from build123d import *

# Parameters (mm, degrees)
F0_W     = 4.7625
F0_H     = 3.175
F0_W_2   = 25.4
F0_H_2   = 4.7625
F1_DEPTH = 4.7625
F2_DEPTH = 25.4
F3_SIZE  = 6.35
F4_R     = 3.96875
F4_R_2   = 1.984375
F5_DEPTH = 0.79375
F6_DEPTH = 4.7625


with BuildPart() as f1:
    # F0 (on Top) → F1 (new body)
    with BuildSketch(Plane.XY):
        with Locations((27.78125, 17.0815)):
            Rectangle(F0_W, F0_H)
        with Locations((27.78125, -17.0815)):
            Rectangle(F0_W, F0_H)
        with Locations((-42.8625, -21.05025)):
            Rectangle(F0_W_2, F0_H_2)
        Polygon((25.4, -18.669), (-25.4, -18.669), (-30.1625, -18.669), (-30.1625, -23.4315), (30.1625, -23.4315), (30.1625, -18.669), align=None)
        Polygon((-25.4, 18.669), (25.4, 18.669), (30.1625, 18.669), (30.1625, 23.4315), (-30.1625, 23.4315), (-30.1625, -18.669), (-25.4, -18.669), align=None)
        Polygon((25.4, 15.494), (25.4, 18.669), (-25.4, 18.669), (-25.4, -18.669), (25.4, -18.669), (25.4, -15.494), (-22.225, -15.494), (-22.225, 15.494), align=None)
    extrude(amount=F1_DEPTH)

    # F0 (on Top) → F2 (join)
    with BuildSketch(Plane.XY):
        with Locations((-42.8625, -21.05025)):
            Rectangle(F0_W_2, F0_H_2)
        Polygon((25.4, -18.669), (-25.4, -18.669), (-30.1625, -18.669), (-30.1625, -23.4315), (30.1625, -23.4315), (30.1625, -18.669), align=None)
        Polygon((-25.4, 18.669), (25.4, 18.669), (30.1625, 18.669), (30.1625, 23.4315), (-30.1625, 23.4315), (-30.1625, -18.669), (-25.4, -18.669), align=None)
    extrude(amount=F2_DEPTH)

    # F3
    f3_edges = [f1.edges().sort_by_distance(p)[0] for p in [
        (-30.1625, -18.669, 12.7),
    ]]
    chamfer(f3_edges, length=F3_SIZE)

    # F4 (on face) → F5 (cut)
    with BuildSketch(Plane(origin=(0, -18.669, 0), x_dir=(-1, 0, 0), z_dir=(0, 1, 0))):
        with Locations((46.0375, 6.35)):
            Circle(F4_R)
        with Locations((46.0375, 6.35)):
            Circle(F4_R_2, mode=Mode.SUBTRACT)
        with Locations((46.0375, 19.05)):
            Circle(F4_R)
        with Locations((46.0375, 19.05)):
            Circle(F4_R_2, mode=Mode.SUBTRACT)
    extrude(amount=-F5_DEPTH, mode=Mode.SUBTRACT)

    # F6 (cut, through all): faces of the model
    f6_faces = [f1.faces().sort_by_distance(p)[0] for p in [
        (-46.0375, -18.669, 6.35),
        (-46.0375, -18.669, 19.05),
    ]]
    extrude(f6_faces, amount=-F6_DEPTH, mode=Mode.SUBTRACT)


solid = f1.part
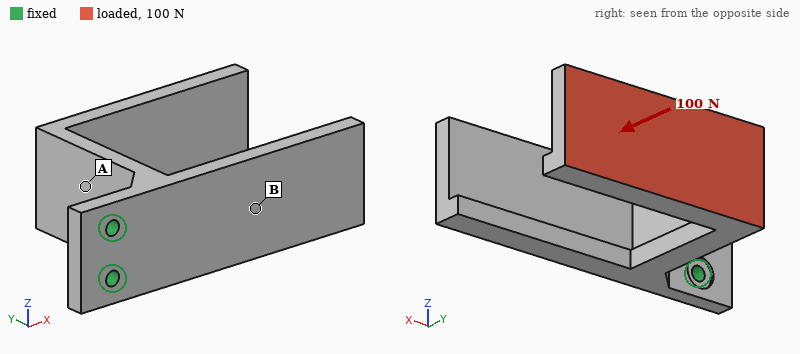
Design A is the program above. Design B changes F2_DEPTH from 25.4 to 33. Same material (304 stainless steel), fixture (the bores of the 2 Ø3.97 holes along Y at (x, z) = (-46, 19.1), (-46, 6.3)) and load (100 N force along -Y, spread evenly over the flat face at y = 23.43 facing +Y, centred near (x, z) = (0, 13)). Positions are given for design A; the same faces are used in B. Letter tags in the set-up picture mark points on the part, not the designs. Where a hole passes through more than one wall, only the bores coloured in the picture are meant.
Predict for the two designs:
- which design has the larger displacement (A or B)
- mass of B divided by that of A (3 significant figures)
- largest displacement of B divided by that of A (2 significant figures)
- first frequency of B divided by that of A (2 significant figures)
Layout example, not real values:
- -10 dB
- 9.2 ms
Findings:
- A
- 1.28
- 0.85
- 0.97
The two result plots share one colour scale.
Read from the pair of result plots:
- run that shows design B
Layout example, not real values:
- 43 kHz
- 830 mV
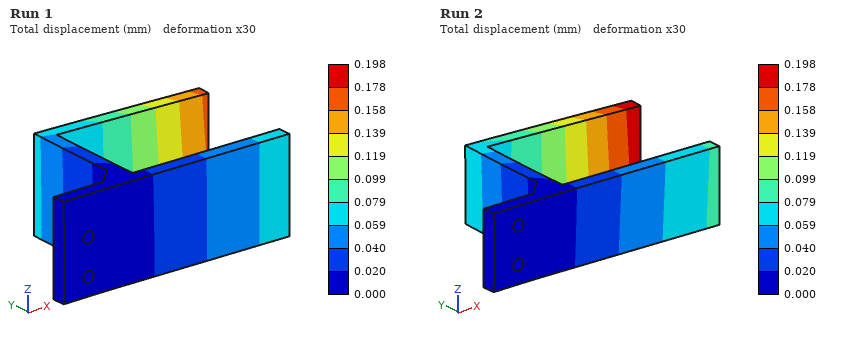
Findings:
- Run 1
